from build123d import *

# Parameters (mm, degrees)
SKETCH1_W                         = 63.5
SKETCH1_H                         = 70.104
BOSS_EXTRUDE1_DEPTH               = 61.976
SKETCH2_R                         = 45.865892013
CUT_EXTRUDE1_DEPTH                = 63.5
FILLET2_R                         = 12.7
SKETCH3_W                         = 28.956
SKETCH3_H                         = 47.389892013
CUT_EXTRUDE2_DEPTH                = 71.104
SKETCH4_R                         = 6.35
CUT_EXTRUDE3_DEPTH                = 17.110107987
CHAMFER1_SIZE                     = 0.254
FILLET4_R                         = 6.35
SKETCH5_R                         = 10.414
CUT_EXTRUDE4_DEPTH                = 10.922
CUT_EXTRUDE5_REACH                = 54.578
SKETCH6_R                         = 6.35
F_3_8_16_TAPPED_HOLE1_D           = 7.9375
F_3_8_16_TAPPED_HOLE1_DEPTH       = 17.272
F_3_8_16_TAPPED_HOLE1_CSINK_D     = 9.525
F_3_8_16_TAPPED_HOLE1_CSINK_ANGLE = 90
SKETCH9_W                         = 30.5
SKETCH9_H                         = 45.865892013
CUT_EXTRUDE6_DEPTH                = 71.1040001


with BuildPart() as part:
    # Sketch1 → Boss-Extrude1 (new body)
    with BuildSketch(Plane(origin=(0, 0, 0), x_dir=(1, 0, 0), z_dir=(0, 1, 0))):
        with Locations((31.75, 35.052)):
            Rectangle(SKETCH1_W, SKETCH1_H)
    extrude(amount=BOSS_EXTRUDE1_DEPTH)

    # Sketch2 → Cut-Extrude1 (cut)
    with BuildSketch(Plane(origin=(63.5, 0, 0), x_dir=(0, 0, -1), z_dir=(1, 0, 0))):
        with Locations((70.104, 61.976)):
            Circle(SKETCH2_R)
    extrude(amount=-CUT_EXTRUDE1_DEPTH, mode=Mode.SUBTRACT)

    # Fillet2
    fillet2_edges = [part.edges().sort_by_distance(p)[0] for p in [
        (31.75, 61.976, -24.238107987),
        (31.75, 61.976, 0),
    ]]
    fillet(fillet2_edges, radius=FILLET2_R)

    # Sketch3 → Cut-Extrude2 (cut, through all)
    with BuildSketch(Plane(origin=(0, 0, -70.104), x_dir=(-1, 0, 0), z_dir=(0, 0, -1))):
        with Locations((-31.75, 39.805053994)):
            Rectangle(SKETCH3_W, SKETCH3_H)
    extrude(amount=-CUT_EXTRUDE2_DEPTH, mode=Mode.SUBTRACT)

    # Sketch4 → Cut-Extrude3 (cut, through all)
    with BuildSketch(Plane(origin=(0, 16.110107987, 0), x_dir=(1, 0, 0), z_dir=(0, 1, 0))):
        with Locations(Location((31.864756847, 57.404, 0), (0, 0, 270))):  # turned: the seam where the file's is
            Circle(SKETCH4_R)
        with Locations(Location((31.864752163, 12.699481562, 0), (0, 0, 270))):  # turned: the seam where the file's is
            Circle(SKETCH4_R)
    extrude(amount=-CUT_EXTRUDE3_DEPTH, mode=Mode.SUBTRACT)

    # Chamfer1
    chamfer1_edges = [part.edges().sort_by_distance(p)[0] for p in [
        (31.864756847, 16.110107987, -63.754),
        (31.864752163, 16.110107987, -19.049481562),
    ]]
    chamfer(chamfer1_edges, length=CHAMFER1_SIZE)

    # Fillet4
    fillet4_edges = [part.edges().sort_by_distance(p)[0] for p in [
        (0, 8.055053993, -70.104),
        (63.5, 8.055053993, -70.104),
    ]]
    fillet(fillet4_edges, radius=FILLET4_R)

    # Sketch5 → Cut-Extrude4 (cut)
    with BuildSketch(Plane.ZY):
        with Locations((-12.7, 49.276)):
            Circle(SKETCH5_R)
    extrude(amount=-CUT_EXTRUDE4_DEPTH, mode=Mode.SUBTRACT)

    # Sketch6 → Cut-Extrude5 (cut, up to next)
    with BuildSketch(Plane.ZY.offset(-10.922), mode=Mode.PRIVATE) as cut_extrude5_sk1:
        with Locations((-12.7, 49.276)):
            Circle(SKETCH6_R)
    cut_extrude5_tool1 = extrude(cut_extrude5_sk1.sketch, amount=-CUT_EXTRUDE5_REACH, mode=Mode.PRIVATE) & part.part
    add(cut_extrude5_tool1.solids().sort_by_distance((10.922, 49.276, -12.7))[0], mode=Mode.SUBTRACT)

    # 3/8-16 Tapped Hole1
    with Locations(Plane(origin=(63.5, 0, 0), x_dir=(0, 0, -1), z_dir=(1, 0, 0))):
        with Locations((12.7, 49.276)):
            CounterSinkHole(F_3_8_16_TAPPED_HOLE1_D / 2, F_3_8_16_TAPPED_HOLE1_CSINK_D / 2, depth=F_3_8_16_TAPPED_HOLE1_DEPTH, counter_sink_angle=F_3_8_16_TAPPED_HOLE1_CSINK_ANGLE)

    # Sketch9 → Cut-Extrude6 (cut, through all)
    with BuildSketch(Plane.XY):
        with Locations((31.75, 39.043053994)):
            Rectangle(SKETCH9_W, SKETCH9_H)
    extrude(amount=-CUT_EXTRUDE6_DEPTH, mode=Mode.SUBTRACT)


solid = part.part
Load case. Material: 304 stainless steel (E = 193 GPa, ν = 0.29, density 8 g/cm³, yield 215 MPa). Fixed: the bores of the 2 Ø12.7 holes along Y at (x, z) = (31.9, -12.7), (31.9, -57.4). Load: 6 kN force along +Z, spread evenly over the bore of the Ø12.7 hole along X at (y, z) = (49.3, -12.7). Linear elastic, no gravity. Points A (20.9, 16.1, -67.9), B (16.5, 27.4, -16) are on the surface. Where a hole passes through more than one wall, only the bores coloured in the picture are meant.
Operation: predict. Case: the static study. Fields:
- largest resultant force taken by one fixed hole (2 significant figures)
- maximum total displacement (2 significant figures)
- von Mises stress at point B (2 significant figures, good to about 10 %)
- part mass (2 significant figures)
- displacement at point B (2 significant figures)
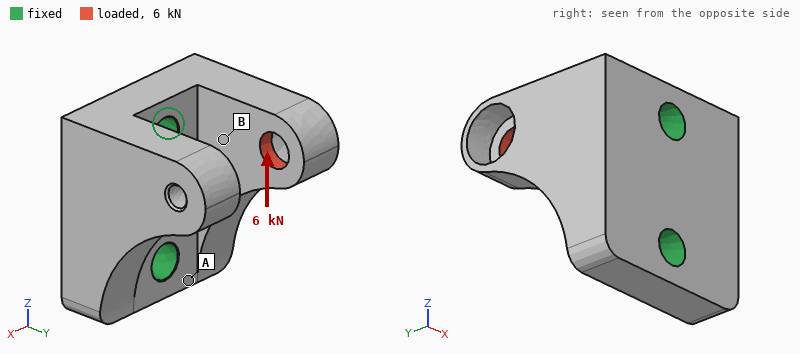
5.9 kN
53 µm
41 MPa
890 g
12 µm
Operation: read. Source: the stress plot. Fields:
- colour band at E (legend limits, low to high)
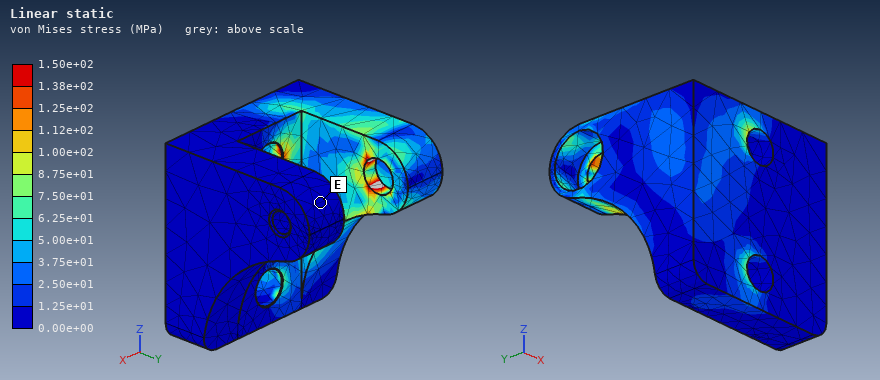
0.00e+00 to 1.25e+01 MPa
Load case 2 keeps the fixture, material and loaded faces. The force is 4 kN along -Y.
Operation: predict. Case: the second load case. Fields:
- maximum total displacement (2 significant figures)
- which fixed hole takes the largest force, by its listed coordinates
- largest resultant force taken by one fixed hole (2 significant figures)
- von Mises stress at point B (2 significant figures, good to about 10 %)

13 µm
(31.9, -12.7)
3.7 kN
22 MPa
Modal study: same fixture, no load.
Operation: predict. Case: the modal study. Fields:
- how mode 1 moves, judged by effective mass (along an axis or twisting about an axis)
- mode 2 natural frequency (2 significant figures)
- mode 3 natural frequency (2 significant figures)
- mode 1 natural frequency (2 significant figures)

along X
4900 Hz
7500 Hz
4100 Hz
